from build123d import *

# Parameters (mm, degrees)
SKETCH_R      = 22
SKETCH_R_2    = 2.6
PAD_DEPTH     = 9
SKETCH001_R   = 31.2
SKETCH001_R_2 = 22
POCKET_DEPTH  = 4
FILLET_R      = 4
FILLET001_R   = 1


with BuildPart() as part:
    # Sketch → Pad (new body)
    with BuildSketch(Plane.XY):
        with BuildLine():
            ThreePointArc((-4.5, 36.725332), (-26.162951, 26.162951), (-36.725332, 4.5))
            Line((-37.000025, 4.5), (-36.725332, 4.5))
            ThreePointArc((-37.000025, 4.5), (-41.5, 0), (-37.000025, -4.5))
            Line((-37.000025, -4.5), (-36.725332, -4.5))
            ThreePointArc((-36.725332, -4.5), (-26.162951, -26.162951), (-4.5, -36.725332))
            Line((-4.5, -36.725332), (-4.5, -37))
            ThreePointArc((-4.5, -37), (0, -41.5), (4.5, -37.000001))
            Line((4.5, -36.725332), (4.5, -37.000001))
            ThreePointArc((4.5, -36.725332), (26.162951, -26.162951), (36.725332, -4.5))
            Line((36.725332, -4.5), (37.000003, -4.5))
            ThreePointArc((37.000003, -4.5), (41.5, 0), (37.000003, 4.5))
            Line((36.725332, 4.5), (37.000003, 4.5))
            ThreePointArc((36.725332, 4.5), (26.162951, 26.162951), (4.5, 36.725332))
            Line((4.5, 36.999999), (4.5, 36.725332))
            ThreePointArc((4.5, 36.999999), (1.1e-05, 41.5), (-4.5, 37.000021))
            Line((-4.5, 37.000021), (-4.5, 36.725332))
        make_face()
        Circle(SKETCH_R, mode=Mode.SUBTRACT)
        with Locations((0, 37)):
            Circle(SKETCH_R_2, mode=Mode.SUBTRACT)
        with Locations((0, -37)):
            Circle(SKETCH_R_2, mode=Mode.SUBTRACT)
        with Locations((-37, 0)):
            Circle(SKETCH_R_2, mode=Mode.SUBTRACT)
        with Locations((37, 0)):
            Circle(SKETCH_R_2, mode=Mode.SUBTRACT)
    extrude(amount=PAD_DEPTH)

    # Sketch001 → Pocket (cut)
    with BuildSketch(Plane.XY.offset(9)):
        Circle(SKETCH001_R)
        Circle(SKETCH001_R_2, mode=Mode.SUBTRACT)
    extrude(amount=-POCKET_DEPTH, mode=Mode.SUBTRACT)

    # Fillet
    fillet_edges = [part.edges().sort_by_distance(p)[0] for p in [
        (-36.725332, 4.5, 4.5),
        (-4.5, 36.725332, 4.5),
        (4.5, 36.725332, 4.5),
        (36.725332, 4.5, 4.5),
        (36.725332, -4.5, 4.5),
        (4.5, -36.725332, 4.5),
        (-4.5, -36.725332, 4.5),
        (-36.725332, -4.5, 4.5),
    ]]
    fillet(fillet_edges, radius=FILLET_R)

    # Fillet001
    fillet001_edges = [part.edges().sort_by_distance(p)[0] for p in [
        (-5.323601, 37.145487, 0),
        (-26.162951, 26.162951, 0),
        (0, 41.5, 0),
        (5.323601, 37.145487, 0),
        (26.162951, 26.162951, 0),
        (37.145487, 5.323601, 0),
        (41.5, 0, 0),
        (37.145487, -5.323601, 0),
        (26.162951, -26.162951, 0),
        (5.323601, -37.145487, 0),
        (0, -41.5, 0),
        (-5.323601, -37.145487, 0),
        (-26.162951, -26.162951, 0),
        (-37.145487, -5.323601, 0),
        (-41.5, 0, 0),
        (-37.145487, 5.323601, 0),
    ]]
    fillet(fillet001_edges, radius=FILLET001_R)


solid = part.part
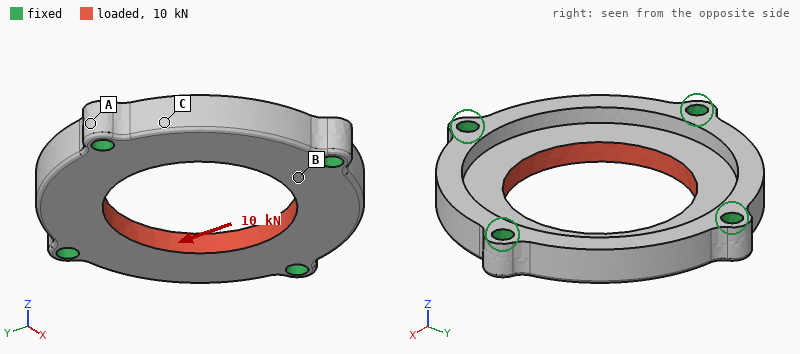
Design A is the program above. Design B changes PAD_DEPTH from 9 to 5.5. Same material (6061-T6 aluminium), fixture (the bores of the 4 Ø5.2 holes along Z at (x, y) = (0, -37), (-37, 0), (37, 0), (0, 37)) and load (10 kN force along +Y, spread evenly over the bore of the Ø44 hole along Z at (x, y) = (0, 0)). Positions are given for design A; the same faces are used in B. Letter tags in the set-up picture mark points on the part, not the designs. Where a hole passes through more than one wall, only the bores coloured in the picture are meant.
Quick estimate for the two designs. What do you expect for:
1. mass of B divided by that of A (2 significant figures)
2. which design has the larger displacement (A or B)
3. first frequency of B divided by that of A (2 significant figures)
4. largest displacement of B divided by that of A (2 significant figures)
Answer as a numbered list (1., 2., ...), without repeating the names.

1. 0.76
2. B
3. 0.69
4. 1.1
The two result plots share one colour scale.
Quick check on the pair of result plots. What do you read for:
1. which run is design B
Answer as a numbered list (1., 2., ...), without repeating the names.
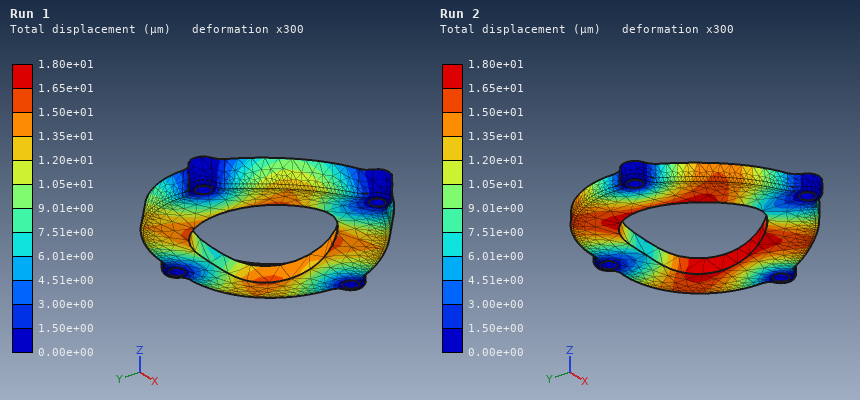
1. Run 2
